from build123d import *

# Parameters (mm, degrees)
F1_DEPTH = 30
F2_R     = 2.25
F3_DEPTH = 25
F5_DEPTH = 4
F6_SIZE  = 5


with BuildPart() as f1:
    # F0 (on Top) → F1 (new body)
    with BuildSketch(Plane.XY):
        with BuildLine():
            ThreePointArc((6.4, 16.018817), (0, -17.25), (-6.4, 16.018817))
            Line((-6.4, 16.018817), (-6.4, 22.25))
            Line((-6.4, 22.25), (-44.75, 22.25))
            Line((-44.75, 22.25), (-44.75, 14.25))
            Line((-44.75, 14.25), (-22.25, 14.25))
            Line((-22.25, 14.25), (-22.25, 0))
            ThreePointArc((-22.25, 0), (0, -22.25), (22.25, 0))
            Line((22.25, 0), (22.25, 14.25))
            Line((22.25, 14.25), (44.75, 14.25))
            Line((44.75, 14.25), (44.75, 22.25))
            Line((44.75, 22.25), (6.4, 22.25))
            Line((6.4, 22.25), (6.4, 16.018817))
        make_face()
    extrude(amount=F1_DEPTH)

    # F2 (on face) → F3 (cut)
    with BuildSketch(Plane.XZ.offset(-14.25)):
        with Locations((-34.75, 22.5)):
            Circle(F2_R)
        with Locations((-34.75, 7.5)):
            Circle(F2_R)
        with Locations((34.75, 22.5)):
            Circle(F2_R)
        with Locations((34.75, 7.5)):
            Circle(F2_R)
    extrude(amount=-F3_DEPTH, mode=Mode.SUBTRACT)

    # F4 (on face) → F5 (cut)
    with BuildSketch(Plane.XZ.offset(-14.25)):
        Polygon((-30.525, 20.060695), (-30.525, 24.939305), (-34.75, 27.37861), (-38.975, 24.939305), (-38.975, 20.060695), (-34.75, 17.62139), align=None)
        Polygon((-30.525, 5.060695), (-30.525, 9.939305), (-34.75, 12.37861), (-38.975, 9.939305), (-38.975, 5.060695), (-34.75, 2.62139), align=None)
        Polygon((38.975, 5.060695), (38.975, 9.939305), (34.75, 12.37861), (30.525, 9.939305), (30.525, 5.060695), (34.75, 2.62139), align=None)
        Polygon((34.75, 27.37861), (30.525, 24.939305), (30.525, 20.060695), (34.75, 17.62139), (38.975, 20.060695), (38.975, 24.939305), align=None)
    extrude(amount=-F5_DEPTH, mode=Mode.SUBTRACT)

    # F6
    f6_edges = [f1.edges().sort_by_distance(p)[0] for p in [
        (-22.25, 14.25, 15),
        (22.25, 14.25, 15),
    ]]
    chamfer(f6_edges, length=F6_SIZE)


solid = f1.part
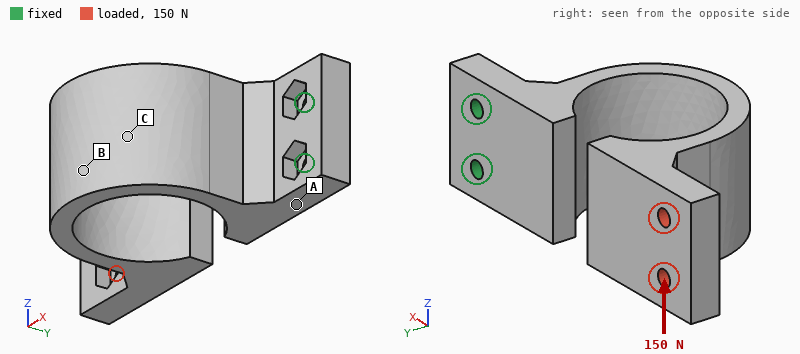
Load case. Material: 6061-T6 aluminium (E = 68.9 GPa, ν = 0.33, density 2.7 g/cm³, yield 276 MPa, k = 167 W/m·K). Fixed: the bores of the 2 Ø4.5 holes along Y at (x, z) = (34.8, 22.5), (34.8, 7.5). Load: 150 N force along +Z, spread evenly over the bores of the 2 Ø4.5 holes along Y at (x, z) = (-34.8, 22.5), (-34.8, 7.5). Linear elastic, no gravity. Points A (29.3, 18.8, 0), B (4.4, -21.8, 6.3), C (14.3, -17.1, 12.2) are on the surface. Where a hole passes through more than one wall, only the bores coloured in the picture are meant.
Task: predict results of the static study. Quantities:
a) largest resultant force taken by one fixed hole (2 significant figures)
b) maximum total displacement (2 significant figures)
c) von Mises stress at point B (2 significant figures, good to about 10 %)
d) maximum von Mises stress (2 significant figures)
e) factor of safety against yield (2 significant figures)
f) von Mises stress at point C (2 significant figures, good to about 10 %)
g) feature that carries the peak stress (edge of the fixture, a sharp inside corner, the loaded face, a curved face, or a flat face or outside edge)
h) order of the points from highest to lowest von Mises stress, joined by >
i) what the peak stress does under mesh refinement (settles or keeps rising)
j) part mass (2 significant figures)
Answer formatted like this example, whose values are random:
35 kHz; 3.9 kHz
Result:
580 N; 0.67 mm; 45 MPa; 64 MPa; 4.3; 56 MPa; a curved face; C > B > A; settles; 90 g
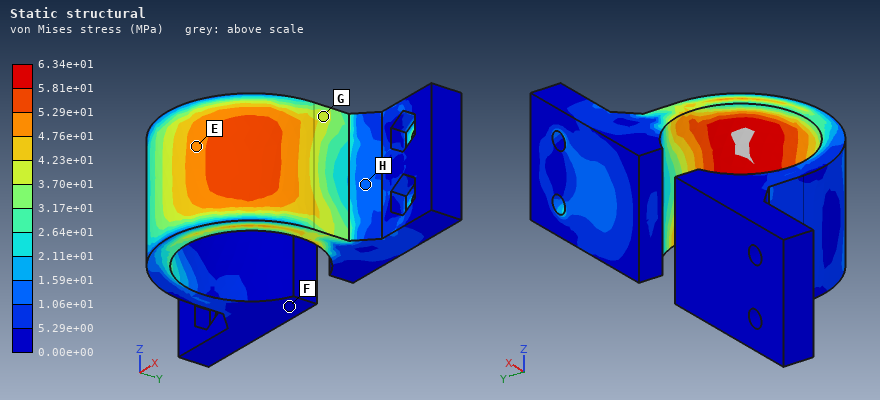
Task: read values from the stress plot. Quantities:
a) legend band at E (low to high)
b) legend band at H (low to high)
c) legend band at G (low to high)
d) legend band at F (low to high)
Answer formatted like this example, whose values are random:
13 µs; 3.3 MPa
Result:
4.76e+01 to 5.29e+01 MPa; 1.06e+01 to 1.59e+01 MPa; 3.70e+01 to 4.23e+01 MPa; 0.00e+00 to 5.29e+00 MPa
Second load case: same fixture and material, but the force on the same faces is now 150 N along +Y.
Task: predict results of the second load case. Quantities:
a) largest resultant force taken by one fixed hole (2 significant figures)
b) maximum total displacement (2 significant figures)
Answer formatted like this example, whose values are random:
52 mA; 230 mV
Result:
82 N; 1.2 mm
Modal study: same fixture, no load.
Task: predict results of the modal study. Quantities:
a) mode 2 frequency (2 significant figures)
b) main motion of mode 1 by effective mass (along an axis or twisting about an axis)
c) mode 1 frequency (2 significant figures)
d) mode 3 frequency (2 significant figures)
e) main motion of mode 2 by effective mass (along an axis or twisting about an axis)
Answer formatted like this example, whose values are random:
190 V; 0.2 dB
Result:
510 Hz; along Y; 360 Hz; 780 Hz; along Z
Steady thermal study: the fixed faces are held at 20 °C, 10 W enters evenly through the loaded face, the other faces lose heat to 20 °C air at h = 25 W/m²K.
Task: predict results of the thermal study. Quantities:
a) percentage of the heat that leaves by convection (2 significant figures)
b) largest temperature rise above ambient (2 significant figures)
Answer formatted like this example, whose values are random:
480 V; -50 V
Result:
42 %; 29 K
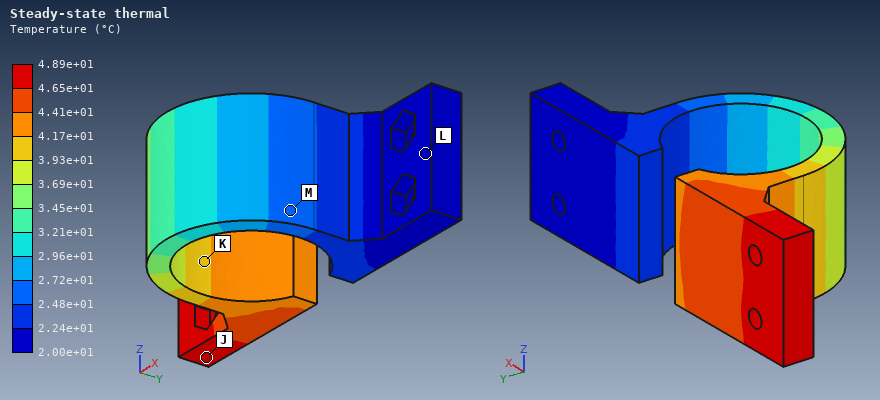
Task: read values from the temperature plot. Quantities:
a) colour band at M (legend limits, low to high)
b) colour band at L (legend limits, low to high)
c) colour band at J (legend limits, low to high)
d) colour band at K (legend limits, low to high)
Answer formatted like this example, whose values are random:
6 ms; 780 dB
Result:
2.48e+01 to 2.72e+01 °C; 2.00e+01 to 2.24e+01 °C; 4.65e+01 to 4.89e+01 °C; 3.93e+01 to 4.17e+01 °C
